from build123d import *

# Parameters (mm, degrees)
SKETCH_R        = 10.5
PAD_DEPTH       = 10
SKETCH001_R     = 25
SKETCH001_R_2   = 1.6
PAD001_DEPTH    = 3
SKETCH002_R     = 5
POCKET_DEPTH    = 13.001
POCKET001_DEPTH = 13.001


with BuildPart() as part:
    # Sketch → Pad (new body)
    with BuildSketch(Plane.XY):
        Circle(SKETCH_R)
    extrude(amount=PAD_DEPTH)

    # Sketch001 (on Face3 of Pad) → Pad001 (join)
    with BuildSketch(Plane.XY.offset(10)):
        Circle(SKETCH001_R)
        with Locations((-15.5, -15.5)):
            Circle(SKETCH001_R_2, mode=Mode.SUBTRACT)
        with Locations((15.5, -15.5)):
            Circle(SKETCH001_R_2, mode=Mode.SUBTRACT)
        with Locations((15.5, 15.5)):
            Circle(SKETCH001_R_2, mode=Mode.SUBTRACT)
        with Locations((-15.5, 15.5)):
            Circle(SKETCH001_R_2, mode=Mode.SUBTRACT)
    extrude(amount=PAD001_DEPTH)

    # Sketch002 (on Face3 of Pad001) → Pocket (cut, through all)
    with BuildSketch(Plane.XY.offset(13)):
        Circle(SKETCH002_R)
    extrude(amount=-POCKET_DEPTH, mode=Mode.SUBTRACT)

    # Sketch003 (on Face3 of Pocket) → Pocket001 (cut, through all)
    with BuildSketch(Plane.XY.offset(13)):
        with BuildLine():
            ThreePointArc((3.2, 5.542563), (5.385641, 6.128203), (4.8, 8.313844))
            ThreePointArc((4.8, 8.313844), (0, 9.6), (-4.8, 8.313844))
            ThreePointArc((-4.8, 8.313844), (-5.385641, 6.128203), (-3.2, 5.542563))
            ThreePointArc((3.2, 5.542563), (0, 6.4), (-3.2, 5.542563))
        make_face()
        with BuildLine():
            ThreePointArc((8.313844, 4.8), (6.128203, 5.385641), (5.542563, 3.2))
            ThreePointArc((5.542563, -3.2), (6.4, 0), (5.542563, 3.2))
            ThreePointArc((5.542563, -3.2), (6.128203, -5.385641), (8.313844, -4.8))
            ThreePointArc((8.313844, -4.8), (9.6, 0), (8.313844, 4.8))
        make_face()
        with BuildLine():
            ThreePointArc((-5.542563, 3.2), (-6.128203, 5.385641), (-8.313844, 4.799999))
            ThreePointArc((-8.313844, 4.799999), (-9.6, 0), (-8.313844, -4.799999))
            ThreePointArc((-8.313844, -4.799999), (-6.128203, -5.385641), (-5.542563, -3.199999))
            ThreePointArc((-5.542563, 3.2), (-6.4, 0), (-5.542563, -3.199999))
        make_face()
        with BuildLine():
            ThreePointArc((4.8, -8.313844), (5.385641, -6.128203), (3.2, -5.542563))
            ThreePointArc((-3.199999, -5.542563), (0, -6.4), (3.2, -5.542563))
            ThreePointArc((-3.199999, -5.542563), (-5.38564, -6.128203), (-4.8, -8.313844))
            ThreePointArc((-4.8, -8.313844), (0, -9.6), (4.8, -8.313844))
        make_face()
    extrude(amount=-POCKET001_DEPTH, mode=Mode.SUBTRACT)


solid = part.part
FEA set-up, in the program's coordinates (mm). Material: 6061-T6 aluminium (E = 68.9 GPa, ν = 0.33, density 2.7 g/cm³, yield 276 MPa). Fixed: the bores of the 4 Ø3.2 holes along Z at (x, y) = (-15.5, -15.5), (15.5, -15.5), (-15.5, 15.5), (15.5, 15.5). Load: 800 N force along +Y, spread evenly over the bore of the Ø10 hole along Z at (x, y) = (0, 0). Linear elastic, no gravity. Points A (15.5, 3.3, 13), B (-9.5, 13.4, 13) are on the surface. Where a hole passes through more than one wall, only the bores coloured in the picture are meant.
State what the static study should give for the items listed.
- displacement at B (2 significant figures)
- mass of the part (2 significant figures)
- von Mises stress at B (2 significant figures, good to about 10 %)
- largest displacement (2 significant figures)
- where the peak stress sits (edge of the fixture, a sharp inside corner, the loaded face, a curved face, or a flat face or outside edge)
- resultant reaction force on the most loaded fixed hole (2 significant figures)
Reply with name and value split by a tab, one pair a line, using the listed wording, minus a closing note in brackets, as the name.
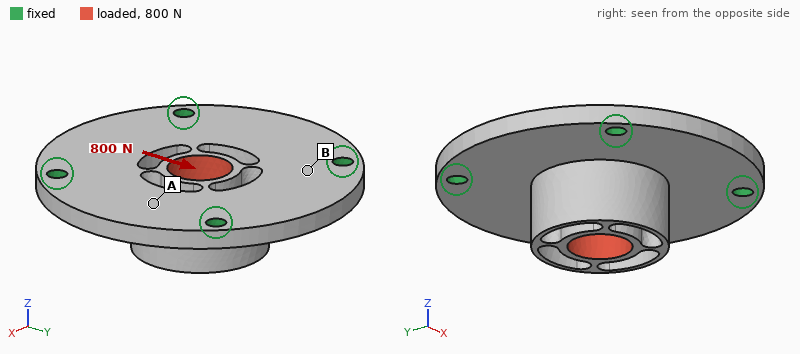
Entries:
displacement at B	3.4 µm
mass of the part	17 g
von Mises stress at B	9.9 MPa
largest displacement	20 µm
where the peak stress sits	a curved face
resultant reaction force on the most loaded fixed hole	230 N
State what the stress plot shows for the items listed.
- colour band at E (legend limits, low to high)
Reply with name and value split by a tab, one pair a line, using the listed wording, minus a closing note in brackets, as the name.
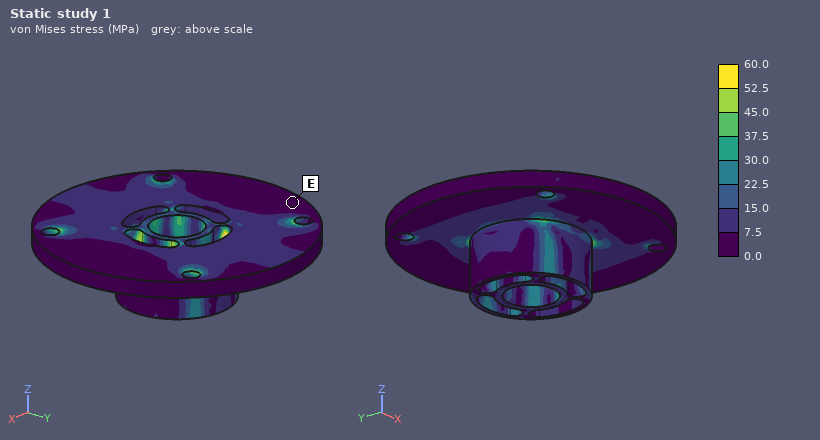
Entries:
colour band at E	0.0 to 7.5 MPa
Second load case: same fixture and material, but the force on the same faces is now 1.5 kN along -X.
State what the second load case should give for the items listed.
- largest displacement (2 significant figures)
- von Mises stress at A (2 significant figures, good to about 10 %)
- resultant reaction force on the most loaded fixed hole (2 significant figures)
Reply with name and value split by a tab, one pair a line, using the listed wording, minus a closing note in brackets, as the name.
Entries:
largest displacement	37 µm
von Mises stress at A	15 MPa
resultant reaction force on the most loaded fixed hole	420 N
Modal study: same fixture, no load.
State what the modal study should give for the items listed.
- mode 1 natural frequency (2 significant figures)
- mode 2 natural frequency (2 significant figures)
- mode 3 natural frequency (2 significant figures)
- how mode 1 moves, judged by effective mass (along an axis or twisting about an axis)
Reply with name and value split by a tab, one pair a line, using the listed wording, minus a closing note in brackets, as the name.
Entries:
mode 1 natural frequency	11 kHz
mode 2 natural frequency	13 kHz
mode 3 natural frequency	13 kHz
how mode 1 moves, judged by effective mass	along Z
